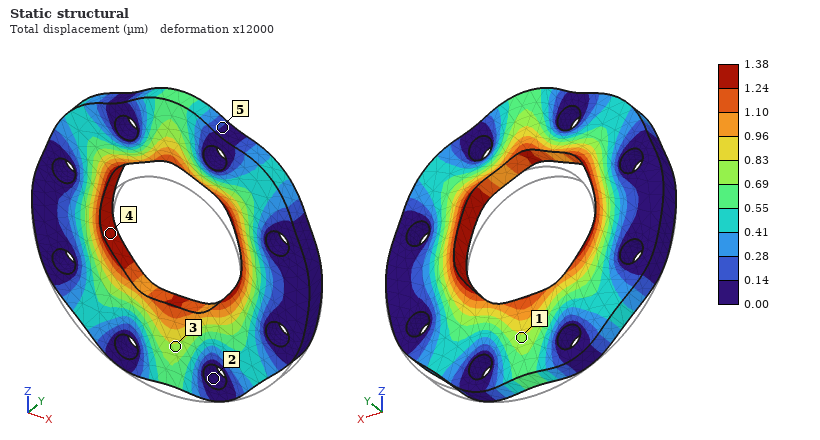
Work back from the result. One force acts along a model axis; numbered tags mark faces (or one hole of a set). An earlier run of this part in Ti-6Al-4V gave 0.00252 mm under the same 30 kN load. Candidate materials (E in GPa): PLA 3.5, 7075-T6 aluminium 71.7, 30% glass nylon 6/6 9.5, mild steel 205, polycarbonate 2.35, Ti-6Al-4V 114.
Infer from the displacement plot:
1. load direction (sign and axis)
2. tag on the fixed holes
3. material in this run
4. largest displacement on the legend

+Z
2
mild steel
1.38 µm
